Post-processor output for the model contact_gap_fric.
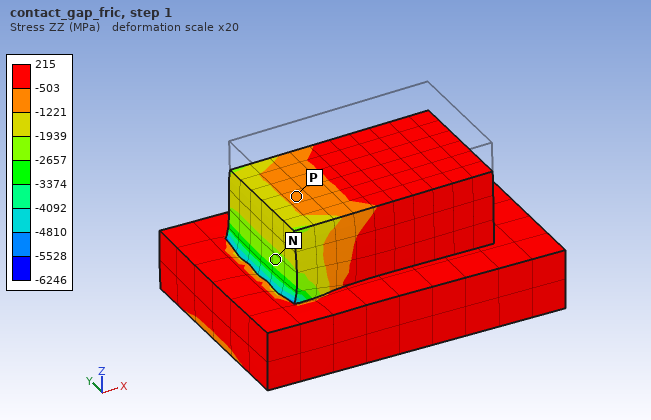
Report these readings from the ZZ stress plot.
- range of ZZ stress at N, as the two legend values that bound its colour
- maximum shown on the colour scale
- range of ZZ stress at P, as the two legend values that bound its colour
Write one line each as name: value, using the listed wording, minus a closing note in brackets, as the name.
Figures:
range of ZZ stress at N, as the two legend values that bound its colour: -2657 to -1939 MPa
maximum shown on the colour scale: 215 MPa
range of ZZ stress at P, as the two legend values that bound its colour: -1221 to -503 MPa
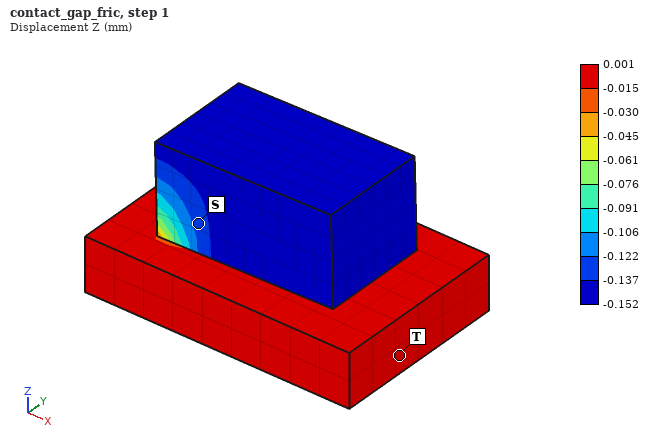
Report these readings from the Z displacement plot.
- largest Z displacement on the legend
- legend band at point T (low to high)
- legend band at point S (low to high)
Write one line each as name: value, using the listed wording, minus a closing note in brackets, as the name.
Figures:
largest Z displacement on the legend: 0.001 mm
legend band at point T: -0.015 to 0.001 mm
legend band at point S: -0.137 to -0.122 mm
